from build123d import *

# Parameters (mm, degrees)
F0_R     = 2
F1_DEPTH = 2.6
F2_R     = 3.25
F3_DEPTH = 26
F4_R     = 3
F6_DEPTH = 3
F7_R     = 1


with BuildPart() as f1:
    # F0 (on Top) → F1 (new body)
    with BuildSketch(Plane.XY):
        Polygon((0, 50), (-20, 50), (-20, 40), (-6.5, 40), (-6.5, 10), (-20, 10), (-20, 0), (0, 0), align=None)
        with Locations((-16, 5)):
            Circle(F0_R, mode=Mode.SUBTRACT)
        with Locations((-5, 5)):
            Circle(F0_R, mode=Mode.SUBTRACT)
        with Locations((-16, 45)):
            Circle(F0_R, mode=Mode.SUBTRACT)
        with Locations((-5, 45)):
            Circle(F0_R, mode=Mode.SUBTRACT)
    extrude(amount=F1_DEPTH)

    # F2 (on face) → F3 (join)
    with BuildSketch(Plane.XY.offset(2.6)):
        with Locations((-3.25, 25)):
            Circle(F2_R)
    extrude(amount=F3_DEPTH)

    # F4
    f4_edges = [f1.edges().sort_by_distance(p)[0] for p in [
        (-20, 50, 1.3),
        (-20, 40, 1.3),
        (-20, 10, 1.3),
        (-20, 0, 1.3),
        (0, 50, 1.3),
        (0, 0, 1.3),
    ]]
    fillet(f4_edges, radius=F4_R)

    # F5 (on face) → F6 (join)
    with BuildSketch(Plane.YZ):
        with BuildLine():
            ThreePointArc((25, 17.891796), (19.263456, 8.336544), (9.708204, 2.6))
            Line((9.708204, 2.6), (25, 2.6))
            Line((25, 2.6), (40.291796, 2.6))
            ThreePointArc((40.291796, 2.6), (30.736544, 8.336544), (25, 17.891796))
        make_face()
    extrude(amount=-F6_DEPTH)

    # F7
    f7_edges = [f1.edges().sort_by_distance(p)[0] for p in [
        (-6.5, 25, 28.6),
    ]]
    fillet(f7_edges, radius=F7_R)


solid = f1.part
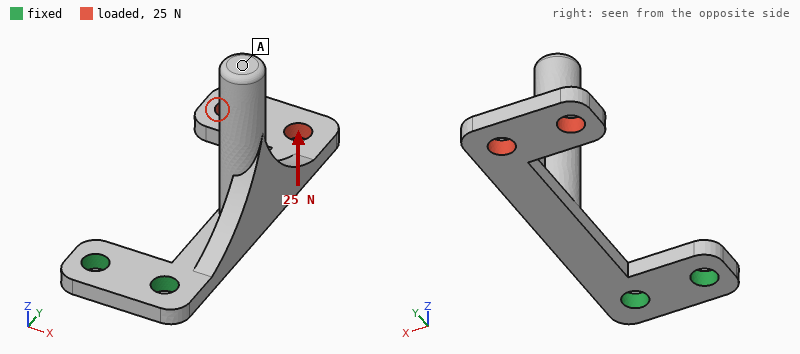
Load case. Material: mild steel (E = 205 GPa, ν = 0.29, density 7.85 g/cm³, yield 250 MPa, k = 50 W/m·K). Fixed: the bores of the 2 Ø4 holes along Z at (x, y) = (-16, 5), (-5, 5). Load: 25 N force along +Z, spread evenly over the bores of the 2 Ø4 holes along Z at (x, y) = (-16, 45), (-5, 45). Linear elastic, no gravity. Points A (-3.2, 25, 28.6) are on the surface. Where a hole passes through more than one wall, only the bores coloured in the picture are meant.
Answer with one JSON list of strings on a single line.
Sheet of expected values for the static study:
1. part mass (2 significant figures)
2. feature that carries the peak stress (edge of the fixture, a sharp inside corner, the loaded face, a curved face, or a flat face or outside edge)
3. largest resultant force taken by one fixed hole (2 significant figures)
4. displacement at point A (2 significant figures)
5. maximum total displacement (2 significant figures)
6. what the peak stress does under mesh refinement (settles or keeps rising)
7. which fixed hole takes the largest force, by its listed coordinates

["20 g", "edge of the fixture", "32 N", "0.095 mm", "0.15 mm", "keeps rising", "(-5, 5)"]
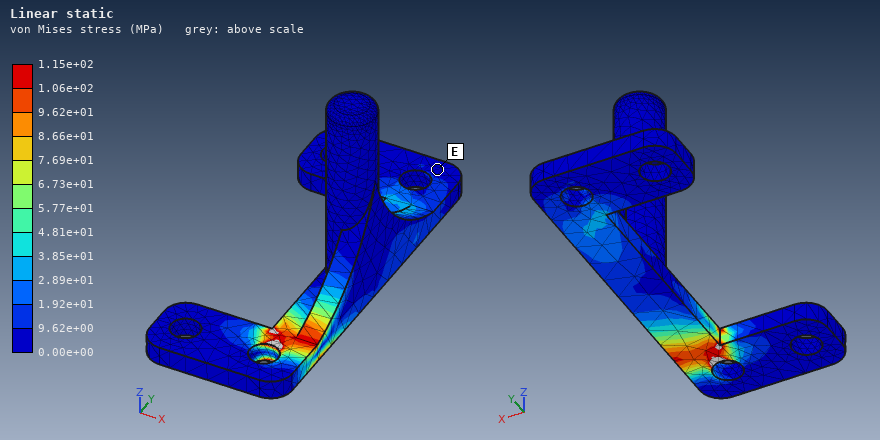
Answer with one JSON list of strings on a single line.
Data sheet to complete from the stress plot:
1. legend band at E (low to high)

["0.00e+00 to 9.62e+00 MPa"]
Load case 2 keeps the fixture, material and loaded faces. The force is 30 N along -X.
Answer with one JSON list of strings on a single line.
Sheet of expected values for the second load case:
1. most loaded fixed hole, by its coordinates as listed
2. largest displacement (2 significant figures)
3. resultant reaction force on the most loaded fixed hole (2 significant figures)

["(-16, 5)", "55 µm", "60 N"]
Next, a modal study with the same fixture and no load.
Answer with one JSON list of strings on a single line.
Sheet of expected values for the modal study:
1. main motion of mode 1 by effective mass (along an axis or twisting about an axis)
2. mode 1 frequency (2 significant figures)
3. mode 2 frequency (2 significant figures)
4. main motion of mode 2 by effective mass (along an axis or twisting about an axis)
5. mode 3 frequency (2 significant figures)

["along Z", "870 Hz", "1600 Hz", "along X", "2100 Hz"]
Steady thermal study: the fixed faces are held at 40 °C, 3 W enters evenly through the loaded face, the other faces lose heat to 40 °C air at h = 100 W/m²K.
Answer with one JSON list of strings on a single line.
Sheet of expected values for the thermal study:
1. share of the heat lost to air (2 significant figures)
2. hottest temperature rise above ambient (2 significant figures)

["84 %", "38 K"]
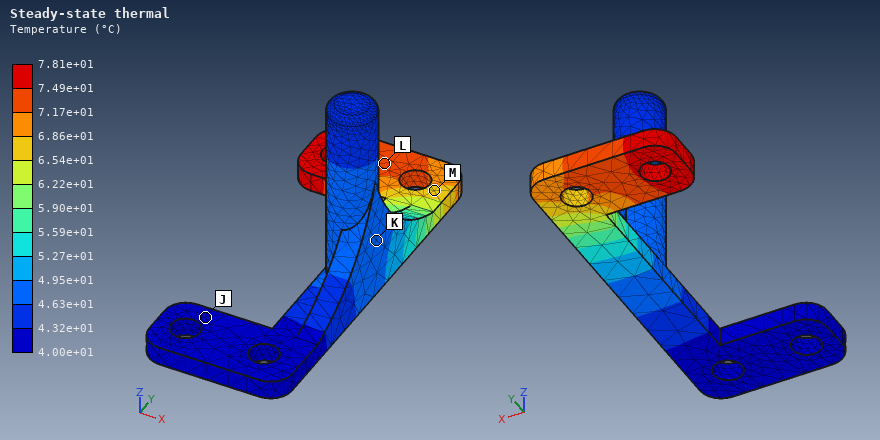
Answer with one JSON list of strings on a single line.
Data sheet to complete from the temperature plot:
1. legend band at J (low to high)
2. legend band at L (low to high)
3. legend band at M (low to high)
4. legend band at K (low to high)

["4.00e+01 to 4.32e+01 °C", "7.17e+01 to 7.49e+01 °C", "6.54e+01 to 6.86e+01 °C", "4.63e+01 to 4.95e+01 °C"]
